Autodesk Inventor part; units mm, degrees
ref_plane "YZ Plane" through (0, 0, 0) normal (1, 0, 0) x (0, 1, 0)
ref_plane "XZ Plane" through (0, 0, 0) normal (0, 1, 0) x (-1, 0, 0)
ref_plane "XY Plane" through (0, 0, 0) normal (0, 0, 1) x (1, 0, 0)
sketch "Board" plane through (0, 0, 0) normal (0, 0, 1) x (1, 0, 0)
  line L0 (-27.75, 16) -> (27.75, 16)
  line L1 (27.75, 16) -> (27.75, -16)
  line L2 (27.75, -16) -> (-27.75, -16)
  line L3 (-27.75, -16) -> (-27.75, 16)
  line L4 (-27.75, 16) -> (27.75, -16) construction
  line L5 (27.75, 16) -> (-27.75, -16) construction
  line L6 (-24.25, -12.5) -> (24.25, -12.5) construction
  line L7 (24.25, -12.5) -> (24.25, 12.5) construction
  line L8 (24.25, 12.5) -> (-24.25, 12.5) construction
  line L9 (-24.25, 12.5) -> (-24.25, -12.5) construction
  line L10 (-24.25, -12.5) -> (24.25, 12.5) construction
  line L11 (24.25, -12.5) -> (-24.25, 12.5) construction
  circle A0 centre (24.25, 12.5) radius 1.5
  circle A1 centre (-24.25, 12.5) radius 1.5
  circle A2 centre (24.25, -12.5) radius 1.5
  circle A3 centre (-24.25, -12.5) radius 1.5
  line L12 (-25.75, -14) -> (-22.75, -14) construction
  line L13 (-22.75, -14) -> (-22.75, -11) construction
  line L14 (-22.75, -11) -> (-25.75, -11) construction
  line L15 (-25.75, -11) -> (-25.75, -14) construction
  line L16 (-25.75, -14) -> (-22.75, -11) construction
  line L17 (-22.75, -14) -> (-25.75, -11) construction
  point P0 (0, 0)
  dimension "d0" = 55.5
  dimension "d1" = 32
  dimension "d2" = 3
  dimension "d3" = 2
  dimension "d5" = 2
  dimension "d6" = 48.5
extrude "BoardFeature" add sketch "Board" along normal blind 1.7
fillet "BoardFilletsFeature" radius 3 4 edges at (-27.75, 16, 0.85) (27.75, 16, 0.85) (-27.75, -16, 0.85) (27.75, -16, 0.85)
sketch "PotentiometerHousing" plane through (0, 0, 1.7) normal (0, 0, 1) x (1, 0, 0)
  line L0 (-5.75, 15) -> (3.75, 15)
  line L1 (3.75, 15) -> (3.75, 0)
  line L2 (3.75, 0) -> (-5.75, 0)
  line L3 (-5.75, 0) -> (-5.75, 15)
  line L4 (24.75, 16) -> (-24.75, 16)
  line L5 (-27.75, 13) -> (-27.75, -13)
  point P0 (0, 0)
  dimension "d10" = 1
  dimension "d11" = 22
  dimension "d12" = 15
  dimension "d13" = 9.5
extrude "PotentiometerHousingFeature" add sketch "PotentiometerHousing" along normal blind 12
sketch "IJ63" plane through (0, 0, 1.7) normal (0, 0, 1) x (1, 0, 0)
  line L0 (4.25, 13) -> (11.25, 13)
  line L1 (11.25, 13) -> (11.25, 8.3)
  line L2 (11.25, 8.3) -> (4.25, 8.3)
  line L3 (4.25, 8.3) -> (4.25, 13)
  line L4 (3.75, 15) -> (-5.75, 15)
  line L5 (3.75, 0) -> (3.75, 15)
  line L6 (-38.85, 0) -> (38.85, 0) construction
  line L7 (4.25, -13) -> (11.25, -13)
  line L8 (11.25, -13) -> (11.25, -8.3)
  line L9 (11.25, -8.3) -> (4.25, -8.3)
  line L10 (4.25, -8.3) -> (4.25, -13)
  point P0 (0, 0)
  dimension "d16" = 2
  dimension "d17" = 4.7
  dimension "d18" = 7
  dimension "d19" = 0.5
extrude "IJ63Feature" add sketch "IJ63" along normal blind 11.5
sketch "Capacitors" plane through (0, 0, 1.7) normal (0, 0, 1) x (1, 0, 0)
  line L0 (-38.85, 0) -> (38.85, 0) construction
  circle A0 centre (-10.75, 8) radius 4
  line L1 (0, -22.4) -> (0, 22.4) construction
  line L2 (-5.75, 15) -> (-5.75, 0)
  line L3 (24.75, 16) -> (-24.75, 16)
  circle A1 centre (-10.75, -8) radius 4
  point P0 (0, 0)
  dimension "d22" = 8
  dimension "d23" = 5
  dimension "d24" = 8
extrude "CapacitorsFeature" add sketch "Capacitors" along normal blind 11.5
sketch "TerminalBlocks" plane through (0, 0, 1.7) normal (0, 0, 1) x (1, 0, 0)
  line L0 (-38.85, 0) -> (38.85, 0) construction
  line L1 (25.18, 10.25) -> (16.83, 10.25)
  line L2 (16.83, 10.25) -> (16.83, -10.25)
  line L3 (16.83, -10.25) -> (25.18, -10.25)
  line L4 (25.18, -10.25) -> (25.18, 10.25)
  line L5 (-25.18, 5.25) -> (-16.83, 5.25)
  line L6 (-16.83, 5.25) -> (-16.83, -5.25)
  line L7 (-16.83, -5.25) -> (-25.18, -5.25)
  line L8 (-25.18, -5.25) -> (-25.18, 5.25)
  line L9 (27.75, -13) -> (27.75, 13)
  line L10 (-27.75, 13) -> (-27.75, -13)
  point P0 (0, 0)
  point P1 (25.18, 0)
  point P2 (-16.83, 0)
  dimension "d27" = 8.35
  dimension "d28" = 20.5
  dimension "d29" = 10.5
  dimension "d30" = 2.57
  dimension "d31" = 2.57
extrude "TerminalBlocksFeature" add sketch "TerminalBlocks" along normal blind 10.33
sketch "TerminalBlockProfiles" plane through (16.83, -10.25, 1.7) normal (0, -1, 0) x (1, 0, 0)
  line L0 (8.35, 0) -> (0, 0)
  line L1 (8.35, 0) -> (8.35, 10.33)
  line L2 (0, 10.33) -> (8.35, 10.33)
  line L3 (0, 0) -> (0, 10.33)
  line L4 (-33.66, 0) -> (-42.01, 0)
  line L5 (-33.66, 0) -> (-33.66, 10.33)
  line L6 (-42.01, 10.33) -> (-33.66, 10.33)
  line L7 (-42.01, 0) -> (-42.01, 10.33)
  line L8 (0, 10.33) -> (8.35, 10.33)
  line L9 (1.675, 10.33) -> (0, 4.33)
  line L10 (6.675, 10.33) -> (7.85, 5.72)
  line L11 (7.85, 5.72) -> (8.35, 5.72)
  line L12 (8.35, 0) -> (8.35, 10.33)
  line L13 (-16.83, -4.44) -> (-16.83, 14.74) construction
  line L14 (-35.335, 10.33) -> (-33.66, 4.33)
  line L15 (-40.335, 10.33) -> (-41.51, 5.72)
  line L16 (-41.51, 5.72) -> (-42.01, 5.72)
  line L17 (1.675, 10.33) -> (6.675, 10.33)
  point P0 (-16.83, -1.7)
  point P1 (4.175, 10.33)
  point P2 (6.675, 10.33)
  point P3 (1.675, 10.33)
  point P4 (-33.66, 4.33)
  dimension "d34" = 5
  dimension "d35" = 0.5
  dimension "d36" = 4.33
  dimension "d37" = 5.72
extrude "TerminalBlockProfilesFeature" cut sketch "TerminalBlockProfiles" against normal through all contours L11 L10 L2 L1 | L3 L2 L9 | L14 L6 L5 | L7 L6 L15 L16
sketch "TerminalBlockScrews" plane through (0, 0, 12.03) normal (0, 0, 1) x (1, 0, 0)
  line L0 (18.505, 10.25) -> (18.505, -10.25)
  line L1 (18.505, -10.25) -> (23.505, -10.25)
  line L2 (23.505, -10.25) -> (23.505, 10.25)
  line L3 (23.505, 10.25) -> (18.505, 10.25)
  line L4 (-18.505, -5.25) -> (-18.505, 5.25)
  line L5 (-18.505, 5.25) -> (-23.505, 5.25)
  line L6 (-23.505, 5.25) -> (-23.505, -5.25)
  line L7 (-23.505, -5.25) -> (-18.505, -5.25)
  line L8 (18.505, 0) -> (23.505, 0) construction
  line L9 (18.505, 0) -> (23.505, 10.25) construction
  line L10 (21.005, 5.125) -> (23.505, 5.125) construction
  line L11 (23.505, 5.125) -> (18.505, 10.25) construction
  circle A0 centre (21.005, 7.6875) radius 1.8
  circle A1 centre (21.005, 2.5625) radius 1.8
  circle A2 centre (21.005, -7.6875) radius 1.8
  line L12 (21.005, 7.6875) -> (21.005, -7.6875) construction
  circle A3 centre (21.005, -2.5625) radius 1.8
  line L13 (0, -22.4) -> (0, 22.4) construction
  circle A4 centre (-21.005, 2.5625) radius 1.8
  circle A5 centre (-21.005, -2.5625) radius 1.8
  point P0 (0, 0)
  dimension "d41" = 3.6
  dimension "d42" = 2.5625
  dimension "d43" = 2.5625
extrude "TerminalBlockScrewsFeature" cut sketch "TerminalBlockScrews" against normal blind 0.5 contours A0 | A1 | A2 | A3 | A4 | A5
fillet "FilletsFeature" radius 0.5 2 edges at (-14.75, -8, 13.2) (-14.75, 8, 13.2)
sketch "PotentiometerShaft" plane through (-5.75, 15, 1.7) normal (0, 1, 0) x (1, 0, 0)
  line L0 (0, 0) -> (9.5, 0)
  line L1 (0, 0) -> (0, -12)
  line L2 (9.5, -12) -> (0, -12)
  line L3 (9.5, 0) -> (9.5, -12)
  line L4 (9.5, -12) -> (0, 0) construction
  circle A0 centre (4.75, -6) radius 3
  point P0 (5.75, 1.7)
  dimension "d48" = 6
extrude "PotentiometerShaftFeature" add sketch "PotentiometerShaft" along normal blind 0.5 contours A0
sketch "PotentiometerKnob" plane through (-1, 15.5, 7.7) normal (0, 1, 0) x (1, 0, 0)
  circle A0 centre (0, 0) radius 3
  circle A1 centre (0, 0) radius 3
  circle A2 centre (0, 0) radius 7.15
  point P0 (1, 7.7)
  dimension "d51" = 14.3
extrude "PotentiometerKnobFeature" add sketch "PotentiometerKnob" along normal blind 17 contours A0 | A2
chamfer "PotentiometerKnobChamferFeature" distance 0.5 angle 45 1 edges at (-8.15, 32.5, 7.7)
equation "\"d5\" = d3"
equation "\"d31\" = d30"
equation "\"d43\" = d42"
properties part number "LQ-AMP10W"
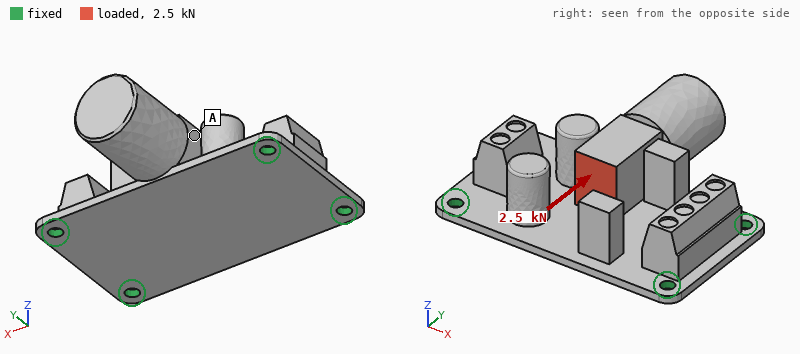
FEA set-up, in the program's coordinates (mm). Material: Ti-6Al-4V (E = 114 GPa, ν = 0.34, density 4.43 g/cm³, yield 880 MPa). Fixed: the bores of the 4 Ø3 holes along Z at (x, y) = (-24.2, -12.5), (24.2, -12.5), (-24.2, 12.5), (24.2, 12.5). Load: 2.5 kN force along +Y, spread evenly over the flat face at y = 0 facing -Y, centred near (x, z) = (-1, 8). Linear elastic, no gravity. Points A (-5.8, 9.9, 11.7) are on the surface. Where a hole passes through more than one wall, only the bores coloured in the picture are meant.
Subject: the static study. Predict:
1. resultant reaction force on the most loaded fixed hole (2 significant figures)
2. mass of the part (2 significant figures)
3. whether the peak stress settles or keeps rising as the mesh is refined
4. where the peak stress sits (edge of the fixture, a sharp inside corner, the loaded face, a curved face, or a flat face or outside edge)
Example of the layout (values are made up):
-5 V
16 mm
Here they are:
1000 N
52 g
keeps rising
edge of the fixture
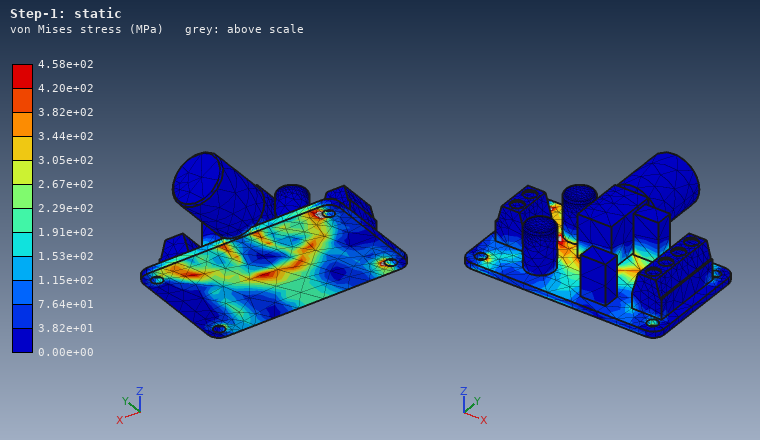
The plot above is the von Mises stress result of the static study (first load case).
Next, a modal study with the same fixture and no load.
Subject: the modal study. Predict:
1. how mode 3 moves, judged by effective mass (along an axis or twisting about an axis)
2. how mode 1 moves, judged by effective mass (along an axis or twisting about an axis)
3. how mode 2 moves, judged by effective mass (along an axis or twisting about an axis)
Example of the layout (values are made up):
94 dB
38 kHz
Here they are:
along X
along Z
along Z
